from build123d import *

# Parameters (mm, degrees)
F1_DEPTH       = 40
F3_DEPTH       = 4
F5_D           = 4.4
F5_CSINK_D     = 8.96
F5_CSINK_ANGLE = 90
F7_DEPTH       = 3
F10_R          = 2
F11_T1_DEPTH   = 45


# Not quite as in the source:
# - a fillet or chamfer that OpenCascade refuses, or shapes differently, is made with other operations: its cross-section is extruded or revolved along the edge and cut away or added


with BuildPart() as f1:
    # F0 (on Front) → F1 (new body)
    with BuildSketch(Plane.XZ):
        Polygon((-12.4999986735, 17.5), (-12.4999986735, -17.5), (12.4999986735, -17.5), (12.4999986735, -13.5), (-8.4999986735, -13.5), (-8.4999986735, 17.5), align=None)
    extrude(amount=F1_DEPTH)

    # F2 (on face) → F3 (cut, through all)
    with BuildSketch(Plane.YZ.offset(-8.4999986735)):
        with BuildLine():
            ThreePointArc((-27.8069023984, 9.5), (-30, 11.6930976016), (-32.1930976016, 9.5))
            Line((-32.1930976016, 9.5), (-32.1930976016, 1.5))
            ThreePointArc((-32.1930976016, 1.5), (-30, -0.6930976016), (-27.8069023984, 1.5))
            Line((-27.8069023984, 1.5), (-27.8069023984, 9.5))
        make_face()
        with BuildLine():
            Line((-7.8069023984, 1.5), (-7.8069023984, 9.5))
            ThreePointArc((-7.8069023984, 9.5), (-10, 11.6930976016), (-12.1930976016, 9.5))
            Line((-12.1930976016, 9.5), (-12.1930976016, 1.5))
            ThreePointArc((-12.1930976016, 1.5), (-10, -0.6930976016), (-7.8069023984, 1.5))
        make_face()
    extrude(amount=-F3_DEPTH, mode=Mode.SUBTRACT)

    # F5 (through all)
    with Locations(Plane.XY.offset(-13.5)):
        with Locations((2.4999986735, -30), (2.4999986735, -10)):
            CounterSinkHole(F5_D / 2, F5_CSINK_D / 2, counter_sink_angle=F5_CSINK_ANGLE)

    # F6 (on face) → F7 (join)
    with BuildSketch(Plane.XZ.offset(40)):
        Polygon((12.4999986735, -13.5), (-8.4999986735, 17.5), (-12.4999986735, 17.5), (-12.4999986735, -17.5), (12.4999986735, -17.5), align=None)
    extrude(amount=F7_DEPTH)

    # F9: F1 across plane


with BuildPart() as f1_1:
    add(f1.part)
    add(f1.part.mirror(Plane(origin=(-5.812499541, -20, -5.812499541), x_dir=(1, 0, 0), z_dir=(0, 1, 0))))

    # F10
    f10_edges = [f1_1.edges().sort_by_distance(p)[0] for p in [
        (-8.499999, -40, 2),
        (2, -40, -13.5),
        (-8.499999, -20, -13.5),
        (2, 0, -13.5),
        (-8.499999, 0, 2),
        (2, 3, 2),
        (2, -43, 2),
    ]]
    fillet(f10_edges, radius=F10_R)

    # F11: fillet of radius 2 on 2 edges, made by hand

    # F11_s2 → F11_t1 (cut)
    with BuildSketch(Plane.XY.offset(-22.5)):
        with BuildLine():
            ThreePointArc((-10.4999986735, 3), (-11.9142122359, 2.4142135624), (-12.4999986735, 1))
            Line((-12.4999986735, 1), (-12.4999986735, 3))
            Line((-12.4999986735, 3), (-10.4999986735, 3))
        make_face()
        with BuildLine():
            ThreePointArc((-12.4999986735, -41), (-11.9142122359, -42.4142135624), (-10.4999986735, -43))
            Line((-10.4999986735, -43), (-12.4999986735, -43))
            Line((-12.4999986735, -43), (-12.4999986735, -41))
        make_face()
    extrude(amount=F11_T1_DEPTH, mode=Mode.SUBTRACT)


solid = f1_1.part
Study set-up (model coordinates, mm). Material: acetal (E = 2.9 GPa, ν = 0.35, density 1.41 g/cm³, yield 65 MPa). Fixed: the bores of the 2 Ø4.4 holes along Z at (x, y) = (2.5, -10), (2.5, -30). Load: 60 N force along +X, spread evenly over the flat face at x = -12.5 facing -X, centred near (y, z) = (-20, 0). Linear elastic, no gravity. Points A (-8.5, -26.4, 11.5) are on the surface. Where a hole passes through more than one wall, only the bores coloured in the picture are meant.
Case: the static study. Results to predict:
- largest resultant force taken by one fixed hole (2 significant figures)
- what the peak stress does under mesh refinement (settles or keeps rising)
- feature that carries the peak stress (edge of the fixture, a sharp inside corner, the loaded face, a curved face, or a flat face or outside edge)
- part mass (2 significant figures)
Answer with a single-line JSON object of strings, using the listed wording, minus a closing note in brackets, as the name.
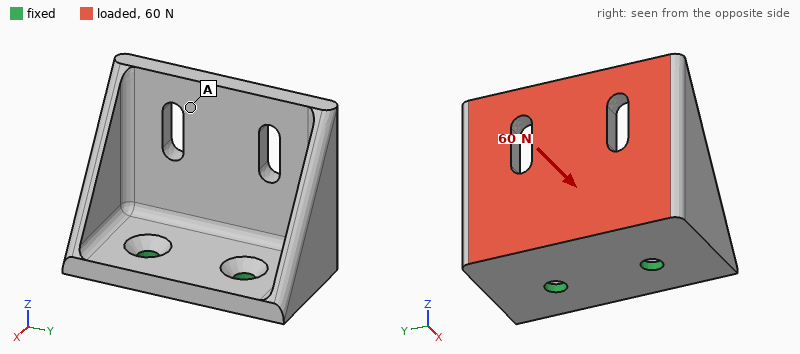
{"largest resultant force taken by one fixed hole": "33 N", "what the peak stress does under mesh refinement": "keeps rising", "feature that carries the peak stress": "edge of the fixture", "part mass": "16 g"}
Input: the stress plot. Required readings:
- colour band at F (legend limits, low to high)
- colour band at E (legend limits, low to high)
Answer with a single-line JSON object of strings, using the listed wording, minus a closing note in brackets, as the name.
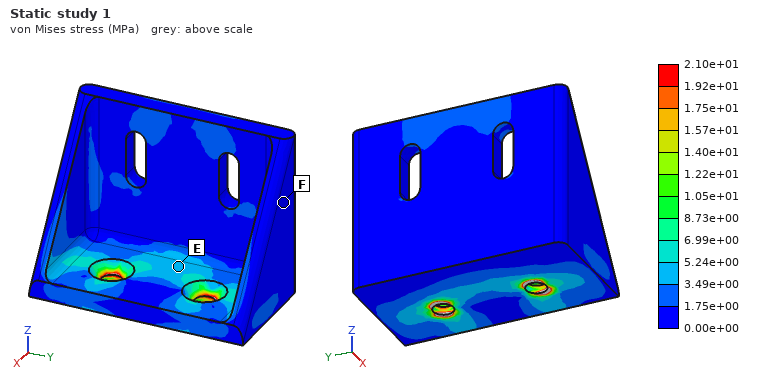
{"colour band at F": "0.00e+00 to 1.75e+00 MPa", "colour band at E": "3.49e+00 to 5.24e+00 MPa"}
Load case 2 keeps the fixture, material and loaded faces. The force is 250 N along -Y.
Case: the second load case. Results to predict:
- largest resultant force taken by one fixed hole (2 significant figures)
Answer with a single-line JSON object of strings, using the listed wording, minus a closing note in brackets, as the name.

{"largest resultant force taken by one fixed hole": "270 N"}
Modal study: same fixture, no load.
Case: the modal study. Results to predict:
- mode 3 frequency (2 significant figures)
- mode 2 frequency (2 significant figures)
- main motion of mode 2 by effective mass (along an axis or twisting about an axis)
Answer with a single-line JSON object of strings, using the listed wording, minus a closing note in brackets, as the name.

{"mode 3 frequency": "1900 Hz", "mode 2 frequency": "890 Hz", "main motion of mode 2 by effective mass": "along Y"}
